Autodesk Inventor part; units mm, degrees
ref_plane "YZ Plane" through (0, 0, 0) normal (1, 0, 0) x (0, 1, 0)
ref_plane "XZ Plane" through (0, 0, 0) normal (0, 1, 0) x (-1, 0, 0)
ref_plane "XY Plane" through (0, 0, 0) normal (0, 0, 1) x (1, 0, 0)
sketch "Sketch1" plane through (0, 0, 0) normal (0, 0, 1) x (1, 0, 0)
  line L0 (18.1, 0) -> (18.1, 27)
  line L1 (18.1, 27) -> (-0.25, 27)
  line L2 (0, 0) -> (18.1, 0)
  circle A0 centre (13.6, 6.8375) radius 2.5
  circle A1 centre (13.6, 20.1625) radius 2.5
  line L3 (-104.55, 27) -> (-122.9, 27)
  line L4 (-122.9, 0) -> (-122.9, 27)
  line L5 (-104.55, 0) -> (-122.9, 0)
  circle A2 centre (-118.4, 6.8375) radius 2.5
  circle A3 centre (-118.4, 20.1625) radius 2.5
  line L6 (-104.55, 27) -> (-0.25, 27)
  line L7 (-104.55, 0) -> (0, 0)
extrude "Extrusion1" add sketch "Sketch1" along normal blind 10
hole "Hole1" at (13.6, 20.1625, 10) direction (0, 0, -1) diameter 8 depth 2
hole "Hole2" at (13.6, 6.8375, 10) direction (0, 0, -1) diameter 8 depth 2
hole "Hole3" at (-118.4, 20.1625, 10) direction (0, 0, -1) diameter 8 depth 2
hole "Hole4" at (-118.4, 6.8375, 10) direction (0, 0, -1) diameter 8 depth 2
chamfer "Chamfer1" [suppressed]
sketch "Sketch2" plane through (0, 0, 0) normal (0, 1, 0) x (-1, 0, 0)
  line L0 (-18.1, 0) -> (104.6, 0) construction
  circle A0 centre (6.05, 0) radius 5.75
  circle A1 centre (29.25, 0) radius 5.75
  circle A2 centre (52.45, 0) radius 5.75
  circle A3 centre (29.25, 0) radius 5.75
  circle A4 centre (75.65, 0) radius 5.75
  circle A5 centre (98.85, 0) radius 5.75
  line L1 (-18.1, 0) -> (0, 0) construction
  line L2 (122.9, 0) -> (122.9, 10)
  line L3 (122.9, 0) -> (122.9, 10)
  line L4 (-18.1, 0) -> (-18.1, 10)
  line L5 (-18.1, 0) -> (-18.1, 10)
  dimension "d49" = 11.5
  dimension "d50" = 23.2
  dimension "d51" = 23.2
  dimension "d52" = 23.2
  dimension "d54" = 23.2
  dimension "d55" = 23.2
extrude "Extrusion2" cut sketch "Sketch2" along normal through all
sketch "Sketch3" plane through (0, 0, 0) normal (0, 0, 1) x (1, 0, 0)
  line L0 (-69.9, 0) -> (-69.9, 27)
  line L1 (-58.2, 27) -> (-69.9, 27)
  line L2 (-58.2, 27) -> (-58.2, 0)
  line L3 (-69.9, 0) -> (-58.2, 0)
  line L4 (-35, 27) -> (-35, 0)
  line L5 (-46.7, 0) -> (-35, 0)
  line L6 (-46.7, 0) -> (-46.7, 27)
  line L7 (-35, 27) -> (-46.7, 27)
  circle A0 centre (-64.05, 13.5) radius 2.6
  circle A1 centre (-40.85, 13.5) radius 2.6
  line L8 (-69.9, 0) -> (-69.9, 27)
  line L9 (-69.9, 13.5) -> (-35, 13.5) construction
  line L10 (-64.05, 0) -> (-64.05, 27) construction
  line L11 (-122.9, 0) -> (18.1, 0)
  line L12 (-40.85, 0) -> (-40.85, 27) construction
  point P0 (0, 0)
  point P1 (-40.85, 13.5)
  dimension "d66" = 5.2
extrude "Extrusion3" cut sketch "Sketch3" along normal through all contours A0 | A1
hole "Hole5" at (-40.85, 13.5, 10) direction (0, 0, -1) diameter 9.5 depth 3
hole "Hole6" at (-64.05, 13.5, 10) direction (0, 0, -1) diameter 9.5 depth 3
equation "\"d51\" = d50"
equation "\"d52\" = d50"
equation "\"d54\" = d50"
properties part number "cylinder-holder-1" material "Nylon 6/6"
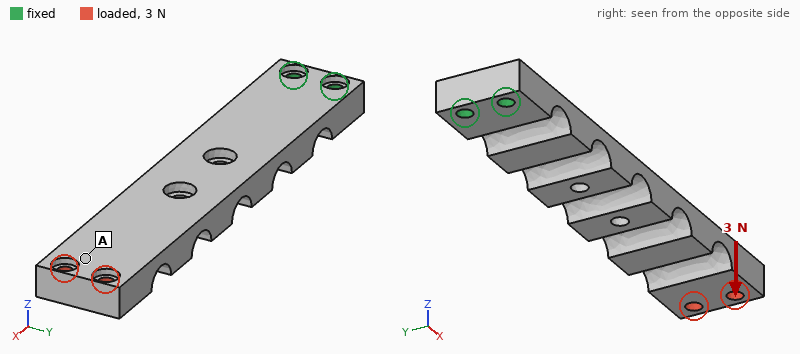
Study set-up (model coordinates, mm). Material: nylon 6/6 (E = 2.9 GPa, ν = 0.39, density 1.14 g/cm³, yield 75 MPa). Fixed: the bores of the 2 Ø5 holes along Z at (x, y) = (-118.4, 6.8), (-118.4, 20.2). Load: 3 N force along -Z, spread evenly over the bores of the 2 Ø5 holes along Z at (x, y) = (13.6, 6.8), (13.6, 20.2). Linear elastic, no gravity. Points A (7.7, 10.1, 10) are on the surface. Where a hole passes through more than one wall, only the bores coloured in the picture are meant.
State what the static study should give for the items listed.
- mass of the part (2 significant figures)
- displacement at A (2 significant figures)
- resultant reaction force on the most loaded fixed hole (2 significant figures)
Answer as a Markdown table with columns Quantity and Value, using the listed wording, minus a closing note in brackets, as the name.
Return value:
| Quantity | Value |
|---|---|
| mass of the part | 33 g |
| displacement at A | 1.4 mm |
| resultant reaction force on the most loaded fixed hole | 1.6 N |
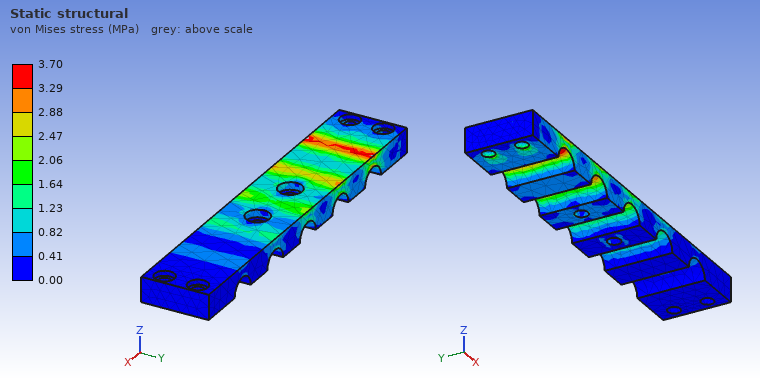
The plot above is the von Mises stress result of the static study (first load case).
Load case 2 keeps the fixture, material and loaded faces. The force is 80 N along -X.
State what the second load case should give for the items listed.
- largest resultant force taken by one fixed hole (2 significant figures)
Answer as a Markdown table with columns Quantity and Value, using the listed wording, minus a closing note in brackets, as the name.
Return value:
| Quantity | Value |
|---|---|
| largest resultant force taken by one fixed hole | 40 N |
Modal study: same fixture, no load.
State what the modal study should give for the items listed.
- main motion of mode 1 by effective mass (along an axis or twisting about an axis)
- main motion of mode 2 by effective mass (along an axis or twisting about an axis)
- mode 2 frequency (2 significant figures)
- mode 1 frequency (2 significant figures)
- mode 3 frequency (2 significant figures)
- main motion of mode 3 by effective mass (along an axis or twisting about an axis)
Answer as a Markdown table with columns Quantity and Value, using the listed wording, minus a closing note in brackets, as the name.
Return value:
| Quantity | Value |
|---|---|
| main motion of mode 1 by effective mass | along Z |
| main motion of mode 2 by effective mass | along Y |
| mode 2 frequency | 300 Hz |
| mode 1 frequency | 76 Hz |
| mode 3 frequency | 480 Hz |
| main motion of mode 3 by effective mass | along Z |
